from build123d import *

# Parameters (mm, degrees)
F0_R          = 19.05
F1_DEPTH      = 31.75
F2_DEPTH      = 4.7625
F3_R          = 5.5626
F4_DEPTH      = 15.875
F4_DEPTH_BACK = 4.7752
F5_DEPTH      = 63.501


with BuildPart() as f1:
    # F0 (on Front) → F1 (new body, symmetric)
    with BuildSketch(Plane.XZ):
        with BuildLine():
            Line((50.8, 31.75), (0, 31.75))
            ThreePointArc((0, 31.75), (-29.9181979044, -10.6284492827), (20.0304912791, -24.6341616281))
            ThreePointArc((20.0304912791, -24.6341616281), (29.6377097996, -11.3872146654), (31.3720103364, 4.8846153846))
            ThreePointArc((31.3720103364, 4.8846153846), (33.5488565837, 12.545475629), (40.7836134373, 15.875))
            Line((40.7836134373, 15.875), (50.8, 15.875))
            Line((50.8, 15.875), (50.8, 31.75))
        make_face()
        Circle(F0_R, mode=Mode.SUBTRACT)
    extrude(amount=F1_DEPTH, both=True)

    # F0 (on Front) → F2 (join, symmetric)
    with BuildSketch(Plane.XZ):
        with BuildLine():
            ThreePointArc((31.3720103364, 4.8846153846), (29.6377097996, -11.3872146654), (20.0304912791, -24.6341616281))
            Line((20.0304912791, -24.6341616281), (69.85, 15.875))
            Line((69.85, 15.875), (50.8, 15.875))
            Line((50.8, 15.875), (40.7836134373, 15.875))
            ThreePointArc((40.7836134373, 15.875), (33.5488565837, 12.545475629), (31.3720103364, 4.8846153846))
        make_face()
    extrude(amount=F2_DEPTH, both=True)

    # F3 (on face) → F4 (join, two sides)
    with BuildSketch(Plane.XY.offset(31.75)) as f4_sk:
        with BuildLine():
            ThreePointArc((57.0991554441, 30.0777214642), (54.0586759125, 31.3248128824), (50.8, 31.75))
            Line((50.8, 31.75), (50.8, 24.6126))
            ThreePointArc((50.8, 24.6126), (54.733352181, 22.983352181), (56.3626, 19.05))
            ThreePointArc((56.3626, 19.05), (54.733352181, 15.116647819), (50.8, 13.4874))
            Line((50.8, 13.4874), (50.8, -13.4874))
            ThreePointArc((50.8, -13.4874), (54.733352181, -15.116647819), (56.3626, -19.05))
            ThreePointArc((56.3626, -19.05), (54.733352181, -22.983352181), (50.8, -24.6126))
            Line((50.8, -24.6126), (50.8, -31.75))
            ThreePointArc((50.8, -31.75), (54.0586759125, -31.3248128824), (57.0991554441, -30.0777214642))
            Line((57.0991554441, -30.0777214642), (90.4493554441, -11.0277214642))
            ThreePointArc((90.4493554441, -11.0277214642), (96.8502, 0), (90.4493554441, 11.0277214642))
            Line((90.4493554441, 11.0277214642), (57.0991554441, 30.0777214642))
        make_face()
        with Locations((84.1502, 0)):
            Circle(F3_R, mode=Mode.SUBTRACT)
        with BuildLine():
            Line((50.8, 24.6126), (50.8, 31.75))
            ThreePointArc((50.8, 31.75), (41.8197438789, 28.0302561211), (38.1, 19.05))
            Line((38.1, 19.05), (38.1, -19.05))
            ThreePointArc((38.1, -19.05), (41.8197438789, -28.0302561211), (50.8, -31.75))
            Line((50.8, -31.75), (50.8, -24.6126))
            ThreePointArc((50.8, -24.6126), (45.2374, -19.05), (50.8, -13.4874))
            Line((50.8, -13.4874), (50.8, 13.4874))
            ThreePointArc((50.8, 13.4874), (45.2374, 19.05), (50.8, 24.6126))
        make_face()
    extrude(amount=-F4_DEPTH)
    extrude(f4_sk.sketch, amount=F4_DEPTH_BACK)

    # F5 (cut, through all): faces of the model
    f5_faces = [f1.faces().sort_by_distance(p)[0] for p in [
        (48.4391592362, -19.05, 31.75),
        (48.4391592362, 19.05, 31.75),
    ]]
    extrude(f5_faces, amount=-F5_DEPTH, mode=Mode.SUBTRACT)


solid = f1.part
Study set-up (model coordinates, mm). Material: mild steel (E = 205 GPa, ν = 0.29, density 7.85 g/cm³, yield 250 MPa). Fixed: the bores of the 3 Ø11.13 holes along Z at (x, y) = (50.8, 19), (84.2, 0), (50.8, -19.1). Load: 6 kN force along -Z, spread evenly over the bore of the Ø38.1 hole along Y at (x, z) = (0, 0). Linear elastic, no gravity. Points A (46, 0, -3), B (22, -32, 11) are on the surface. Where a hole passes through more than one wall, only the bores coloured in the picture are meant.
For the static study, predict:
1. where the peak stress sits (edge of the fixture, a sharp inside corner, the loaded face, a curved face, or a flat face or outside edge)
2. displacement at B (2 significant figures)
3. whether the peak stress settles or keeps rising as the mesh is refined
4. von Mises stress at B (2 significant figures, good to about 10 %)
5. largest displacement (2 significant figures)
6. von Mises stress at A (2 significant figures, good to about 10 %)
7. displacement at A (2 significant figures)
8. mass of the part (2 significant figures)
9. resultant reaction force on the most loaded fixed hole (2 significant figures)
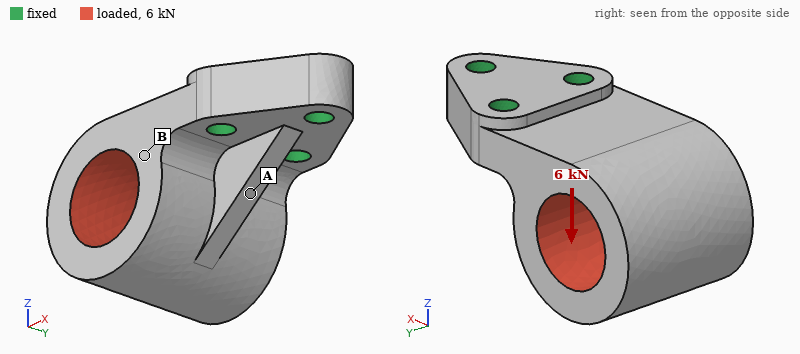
edge of the fixture
13 µm
keeps rising
12 MPa
50 µm
40 MPa
12 µm
1.6 kg
4.3 kN
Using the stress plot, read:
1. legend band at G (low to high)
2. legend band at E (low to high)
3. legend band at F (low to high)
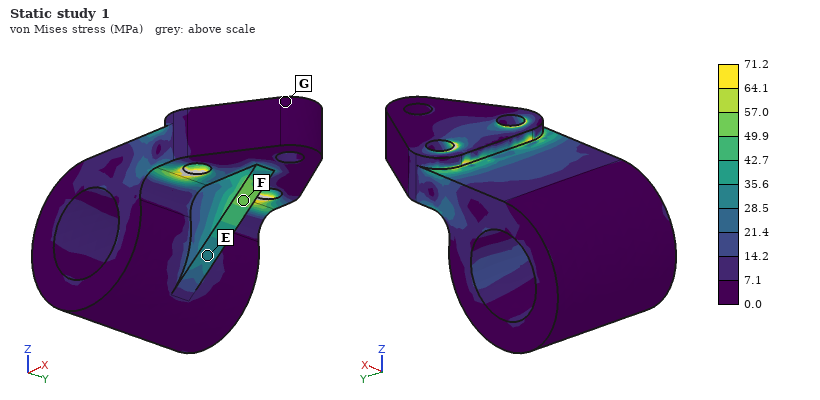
0.0 to 7.1 MPa
28.5 to 35.6 MPa
49.9 to 57.0 MPa
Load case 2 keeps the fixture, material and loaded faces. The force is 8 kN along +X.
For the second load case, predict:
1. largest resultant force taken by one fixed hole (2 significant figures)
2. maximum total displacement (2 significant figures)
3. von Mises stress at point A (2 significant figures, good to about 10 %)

3.2 kN
37 µm
42 MPa
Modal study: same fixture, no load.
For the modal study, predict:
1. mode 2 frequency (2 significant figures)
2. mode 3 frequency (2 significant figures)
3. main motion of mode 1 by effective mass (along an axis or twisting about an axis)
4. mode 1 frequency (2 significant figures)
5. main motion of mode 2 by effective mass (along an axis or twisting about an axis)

3400 Hz
5500 Hz
along Z
1800 Hz
along Y
